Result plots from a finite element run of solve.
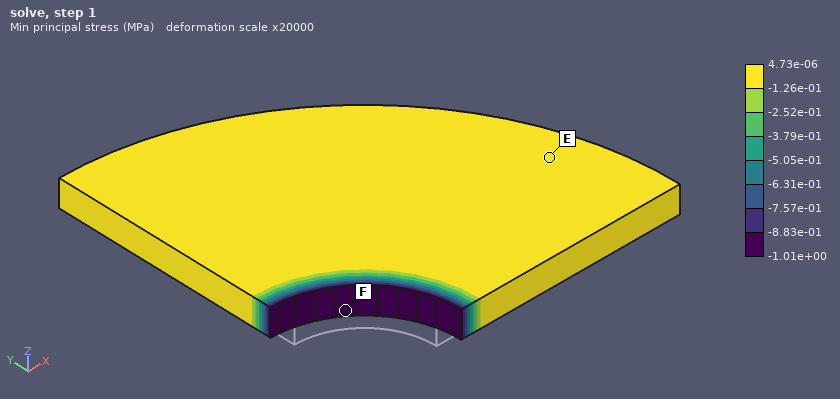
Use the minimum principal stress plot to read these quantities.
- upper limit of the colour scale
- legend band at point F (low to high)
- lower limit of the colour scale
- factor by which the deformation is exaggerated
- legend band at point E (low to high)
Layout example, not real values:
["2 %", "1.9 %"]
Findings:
["4.73e-06 MPa", "-1.01e+00 to -8.83e-01 MPa", "-1.01e+00 MPa", "20000", "-1.26e-01 to 4.73e-06 MPa"]
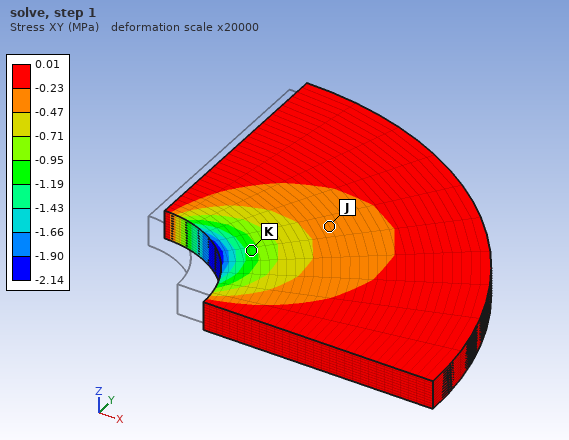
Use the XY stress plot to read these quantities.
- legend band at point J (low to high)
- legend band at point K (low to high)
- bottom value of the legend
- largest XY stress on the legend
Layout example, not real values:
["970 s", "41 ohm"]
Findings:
["-0.47 to -0.23 MPa", "-1.19 to -0.95 MPa", "-2.14 MPa", "0.01 MPa"]
